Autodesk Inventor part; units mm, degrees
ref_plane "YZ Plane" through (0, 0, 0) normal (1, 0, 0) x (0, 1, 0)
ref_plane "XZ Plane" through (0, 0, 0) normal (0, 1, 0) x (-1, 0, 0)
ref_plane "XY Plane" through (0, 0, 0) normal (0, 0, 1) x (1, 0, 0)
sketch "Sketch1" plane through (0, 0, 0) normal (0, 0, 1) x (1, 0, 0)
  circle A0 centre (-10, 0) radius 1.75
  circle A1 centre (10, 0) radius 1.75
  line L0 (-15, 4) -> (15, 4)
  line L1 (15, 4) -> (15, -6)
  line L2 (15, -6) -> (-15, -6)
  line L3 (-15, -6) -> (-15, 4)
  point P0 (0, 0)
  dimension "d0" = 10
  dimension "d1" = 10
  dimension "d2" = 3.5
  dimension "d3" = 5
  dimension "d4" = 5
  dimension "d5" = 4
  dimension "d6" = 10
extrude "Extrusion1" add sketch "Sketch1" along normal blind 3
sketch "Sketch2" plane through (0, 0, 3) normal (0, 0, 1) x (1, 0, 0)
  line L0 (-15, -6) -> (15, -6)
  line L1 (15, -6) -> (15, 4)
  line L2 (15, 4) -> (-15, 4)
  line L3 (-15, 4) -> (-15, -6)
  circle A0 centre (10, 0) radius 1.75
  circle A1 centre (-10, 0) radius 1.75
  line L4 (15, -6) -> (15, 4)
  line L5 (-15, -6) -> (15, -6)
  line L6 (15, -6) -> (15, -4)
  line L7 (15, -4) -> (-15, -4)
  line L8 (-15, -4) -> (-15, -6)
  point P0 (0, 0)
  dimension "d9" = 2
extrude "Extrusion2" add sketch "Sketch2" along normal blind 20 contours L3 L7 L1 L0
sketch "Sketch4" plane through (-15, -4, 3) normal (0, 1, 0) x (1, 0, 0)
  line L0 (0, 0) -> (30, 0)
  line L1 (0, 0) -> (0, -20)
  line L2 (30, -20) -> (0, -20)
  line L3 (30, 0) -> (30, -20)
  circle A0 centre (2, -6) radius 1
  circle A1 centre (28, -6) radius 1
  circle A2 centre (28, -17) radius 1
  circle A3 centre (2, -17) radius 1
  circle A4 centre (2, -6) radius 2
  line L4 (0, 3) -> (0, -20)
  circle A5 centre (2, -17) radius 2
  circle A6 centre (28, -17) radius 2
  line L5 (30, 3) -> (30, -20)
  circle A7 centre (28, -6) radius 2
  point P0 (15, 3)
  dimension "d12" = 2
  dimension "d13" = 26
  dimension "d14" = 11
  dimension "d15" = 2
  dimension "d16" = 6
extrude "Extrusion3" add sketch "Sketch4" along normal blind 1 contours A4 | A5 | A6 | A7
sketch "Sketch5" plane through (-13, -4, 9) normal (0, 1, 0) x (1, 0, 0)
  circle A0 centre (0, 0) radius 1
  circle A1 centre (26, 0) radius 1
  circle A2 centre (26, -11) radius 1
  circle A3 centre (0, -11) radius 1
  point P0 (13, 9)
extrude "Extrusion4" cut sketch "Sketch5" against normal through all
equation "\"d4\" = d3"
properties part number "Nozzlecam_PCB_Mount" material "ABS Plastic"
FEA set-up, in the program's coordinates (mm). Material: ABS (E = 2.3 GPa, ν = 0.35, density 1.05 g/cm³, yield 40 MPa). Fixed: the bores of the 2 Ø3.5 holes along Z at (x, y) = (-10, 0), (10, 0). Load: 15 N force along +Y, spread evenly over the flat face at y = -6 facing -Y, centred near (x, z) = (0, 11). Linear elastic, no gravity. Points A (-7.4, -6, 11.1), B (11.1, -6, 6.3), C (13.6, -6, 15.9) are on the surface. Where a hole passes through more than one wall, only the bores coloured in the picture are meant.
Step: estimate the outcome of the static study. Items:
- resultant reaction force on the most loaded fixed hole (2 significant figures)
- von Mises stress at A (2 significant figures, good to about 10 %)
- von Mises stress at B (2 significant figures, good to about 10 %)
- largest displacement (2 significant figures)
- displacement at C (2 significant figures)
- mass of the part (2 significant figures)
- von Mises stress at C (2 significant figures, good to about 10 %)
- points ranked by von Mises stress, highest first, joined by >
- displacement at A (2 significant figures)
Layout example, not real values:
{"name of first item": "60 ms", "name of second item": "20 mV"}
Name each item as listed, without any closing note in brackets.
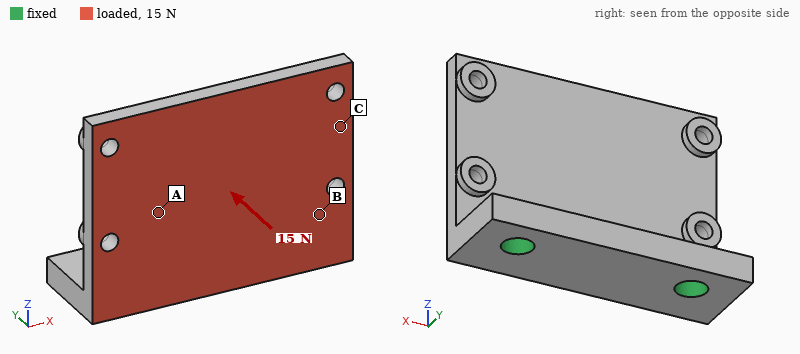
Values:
{"resultant reaction force on the most loaded fixed hole": "7.6 N", "von Mises stress at A": "2.1 MPa", "von Mises stress at B": "4.4 MPa", "largest displacement": "0.40 mm", "displacement at C": "0.23 mm", "mass of the part": "2.2 g", "von Mises stress at C": "0.89 MPa", "points ranked by von Mises stress, highest first, joined by >": "B > A > C", "displacement at A": "0.13 mm"}
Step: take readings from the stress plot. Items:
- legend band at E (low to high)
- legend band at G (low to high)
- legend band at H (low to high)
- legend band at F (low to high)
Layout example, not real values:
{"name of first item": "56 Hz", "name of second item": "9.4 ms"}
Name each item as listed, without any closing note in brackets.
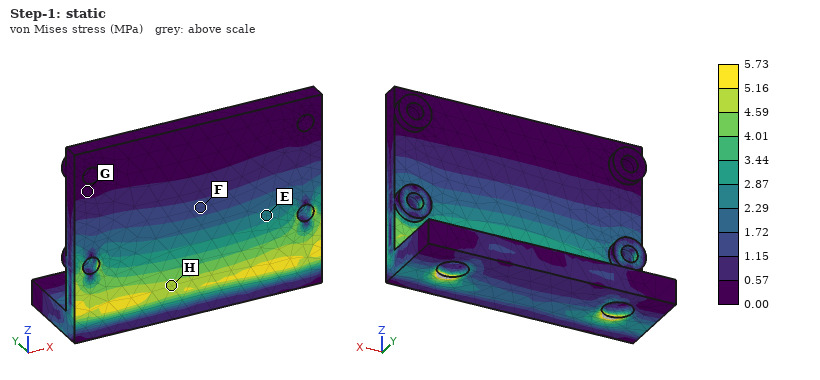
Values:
{"legend band at E": "2.29 to 2.87 MPa", "legend band at G": "0.00 to 0.57 MPa", "legend band at H": "4.59 to 5.16 MPa", "legend band at F": "1.15 to 1.72 MPa"}
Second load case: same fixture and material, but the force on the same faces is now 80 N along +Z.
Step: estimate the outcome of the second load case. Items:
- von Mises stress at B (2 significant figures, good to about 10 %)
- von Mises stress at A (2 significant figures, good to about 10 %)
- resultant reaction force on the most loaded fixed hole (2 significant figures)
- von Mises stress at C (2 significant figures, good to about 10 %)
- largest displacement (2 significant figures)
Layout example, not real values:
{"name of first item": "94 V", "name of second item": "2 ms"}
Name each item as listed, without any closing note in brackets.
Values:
{"von Mises stress at B": "4.3 MPa", "von Mises stress at A": "2.7 MPa", "resultant reaction force on the most loaded fixed hole": "40 N", "von Mises stress at C": "1.6 MPa", "largest displacement": "0.41 mm"}
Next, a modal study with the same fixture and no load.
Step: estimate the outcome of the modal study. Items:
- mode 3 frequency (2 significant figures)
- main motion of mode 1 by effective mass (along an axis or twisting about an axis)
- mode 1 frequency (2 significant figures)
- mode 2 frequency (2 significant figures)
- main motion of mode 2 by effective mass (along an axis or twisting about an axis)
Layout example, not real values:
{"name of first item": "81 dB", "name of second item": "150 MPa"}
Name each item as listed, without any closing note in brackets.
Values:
{"mode 3 frequency": "4600 Hz", "main motion of mode 1 by effective mass": "along Y", "mode 1 frequency": "1000 Hz", "mode 2 frequency": "1900 Hz", "main motion of mode 2 by effective mass": "twisting about Z"}
